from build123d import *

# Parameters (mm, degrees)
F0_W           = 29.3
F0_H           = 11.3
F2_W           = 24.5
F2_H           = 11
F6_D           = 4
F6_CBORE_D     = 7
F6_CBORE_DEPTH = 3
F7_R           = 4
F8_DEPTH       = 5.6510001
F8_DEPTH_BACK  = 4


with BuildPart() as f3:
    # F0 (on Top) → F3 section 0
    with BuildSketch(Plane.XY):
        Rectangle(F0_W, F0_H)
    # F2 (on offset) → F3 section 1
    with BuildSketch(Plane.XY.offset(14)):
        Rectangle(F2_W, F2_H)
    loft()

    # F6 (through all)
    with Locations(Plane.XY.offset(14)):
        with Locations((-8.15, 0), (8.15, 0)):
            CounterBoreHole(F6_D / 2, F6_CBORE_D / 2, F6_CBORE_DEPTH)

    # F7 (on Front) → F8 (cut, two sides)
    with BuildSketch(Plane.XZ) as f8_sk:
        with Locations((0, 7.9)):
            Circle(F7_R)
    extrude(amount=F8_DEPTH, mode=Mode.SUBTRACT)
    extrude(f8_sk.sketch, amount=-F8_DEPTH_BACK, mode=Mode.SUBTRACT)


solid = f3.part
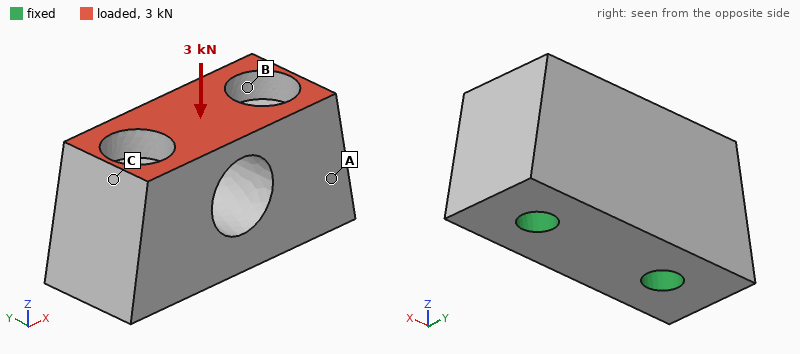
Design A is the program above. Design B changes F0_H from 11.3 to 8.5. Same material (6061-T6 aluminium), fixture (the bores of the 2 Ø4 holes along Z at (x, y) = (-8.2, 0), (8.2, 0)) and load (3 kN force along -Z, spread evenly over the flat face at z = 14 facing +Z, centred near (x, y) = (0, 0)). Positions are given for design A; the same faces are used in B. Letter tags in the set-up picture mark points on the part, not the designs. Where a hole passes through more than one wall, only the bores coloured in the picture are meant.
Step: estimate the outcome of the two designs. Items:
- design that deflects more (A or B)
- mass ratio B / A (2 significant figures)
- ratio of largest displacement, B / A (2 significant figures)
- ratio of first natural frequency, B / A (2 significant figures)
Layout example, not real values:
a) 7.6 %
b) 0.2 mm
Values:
a) B
b) 0.84
c) 1.1
d) 0.97
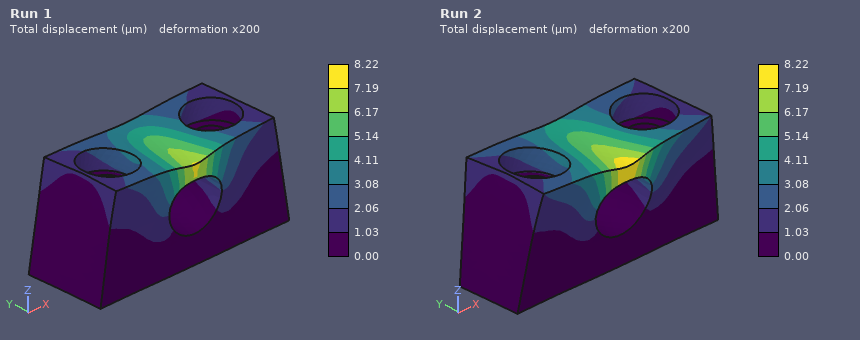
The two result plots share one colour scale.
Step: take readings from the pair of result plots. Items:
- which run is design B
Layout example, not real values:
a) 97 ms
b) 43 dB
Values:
a) Run 2
